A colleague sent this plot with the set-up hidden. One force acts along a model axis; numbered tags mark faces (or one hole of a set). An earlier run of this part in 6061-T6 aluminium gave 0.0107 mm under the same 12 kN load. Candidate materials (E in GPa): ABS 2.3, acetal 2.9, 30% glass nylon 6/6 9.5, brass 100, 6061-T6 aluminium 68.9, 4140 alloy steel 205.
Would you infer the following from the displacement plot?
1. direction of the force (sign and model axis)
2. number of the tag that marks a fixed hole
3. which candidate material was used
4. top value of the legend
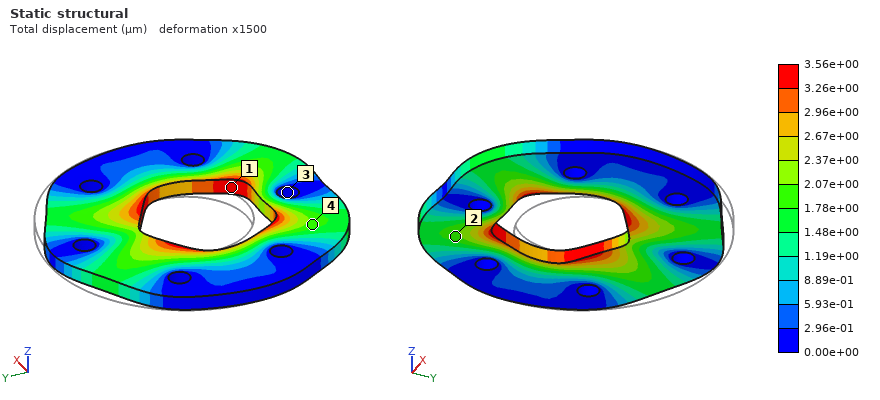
-Y
3
4140 alloy steel
3.56e+00 µm
